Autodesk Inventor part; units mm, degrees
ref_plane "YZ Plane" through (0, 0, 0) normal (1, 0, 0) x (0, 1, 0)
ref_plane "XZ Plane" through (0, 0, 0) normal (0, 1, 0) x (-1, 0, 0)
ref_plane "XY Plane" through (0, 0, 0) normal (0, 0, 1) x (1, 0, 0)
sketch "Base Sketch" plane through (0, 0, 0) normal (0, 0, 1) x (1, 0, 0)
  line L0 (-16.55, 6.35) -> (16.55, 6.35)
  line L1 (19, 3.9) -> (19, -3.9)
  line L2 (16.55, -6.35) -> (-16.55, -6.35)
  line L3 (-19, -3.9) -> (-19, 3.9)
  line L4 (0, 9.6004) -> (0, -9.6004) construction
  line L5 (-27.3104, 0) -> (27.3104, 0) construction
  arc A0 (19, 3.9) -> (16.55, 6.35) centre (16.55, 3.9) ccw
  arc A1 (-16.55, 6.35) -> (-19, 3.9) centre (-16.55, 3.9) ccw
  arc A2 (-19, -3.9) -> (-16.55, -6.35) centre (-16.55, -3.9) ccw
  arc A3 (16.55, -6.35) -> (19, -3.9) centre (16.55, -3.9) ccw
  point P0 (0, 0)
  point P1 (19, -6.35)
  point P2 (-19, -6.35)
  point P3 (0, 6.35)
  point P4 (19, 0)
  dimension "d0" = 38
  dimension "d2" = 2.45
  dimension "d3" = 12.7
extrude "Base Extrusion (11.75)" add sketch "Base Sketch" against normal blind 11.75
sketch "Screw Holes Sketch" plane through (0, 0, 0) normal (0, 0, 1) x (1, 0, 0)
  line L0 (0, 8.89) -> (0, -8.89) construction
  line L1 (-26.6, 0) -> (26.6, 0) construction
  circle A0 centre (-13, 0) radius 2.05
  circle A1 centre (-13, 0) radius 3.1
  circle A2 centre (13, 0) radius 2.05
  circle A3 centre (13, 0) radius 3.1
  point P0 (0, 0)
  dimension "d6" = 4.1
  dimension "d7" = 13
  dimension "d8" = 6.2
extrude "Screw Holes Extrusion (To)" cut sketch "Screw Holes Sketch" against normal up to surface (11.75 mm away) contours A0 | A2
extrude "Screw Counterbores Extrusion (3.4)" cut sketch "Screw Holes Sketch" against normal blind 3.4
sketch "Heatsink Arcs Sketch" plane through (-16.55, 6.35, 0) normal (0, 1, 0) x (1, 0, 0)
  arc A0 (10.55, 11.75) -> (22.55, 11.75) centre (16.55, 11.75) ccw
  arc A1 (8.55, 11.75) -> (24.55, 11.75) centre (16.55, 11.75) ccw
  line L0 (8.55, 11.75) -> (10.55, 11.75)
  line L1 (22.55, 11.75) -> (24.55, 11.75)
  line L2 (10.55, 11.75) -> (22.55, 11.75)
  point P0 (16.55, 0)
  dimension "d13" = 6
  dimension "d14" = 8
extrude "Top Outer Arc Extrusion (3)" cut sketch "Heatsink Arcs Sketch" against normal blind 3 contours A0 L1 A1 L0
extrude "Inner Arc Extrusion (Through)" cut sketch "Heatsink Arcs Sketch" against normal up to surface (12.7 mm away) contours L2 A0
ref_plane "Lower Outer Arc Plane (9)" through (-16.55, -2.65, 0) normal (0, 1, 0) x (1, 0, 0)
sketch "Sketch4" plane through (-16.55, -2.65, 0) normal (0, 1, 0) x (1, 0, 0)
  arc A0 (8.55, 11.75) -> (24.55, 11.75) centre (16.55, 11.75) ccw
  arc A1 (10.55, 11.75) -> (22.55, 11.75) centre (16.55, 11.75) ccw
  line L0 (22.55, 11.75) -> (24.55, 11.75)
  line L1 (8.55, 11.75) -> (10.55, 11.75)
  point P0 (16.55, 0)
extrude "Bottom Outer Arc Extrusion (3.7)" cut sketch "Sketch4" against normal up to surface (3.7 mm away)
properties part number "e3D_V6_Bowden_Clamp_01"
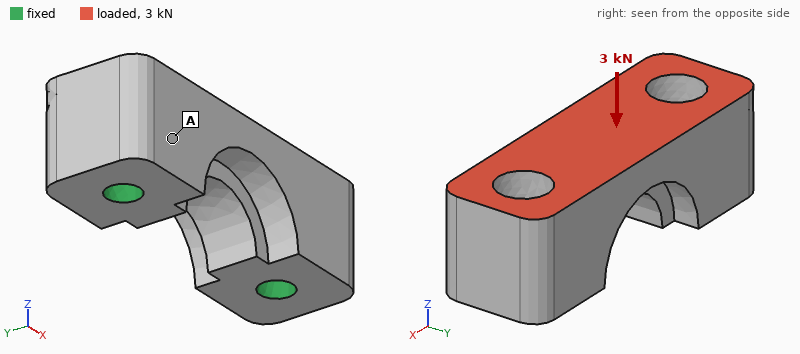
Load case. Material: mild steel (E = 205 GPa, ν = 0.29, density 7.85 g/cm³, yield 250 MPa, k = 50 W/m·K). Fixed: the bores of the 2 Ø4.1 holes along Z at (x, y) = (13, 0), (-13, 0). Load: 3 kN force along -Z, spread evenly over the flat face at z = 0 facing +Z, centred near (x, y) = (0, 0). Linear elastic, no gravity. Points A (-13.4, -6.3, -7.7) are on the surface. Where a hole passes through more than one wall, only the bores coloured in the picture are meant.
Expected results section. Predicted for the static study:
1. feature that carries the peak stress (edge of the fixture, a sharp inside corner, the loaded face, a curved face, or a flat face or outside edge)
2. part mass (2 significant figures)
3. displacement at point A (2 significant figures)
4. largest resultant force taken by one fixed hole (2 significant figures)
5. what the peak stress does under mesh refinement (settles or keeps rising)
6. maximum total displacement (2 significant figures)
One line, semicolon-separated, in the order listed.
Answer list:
edge of the fixture; 33 g; 0.32 µm; 1.6 kN; keeps rising; 1.9 µm
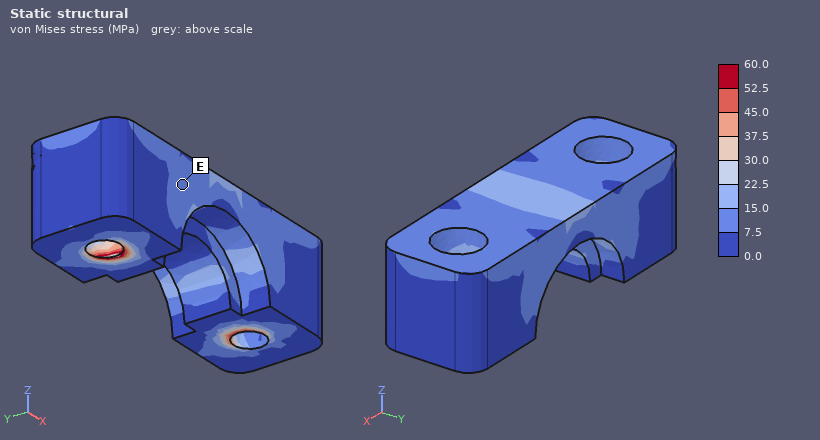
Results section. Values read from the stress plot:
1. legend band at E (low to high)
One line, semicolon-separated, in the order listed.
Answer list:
7.5 to 15.0 MPa
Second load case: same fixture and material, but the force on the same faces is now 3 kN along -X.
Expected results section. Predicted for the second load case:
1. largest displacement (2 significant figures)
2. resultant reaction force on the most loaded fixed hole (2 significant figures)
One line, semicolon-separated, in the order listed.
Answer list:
1.9 µm; 1.6 kN
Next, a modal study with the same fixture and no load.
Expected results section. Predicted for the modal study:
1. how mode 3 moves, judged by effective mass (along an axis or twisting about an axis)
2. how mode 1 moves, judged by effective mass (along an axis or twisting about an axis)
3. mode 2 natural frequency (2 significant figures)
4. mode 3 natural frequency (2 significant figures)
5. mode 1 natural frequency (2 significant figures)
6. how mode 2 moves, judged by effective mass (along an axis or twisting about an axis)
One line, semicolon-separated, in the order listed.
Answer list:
twisting about X; along Y; 52 kHz; 61 kHz; 39 kHz; along Z
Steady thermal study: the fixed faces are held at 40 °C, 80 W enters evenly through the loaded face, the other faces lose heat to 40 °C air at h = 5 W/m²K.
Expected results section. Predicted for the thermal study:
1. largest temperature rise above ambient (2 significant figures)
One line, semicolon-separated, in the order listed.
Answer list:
60 K
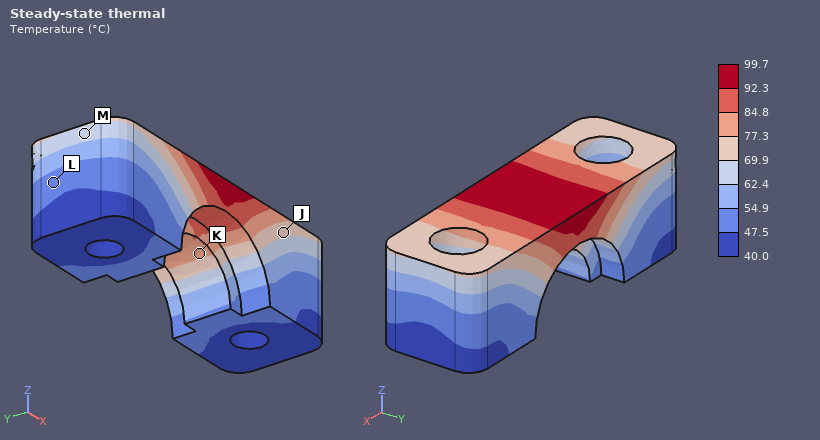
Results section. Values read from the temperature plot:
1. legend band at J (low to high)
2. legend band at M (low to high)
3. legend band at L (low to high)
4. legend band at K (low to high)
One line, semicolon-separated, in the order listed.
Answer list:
69.9 to 77.3 °C; 62.4 to 69.9 °C; 47.5 to 54.9 °C; 77.3 to 84.8 °C
